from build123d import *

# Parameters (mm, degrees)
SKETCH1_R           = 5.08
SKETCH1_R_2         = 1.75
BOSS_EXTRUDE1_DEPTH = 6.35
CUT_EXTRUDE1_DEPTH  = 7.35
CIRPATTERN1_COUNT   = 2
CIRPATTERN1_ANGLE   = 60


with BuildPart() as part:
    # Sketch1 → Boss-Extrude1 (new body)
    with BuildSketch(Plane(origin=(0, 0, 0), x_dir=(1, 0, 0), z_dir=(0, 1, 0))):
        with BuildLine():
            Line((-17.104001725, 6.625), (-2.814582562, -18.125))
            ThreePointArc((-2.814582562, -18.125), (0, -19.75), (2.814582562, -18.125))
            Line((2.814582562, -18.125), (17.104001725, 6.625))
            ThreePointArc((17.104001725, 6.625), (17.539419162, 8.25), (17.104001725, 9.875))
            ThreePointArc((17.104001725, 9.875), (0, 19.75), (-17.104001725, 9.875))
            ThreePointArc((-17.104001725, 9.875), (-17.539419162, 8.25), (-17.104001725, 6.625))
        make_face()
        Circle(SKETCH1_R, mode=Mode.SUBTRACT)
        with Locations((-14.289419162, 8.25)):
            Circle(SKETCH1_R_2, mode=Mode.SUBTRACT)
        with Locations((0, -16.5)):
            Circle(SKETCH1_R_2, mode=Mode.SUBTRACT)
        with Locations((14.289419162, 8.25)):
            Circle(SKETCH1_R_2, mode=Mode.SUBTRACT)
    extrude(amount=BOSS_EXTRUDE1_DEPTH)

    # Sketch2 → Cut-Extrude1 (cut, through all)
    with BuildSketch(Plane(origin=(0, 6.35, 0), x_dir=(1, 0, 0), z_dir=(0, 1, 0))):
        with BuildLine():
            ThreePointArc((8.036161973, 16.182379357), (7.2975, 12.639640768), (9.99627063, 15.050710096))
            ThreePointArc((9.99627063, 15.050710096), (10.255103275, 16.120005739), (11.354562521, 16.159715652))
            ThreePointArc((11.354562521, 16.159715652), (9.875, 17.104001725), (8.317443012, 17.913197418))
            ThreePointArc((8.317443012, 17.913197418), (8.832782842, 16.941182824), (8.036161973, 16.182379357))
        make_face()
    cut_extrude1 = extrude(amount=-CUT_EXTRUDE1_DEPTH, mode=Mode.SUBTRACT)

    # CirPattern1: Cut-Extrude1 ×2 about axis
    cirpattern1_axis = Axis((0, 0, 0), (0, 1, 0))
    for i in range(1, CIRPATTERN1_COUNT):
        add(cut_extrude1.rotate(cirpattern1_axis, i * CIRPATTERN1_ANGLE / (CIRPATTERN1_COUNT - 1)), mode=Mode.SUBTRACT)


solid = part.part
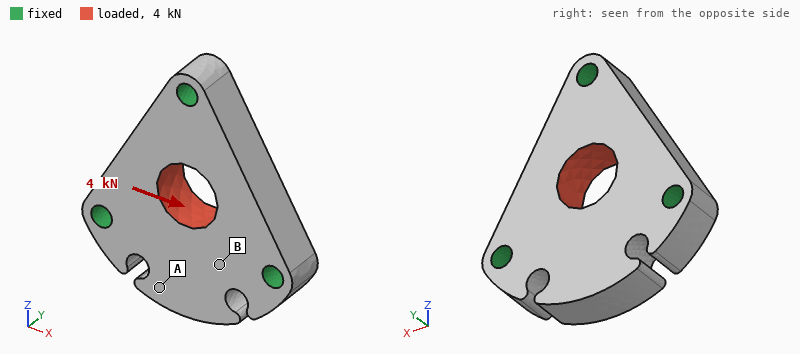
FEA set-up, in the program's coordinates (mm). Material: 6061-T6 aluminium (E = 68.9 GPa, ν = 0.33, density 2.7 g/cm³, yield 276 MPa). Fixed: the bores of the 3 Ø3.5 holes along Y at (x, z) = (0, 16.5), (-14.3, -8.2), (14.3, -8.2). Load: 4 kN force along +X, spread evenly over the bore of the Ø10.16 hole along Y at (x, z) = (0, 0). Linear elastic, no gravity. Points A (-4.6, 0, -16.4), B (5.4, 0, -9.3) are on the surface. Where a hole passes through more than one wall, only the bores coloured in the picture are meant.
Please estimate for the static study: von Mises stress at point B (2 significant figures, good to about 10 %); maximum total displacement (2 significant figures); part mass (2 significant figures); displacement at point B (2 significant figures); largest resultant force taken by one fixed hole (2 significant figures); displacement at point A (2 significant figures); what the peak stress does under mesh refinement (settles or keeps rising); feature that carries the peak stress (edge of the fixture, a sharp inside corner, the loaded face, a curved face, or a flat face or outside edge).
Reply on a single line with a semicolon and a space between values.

21 MPa; 12 µm; 12 g; 2.5 µm; 1.6 kN; 2.8 µm; keeps rising; edge of the fixture
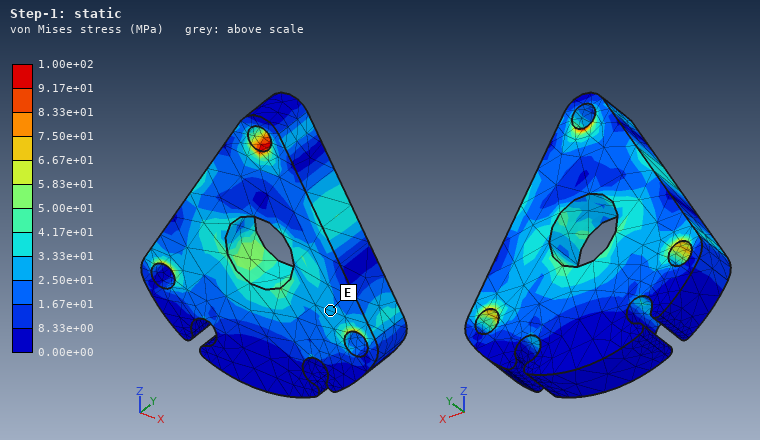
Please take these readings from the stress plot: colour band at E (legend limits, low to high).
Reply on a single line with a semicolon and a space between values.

2.50e+01 to 3.33e+01 MPa
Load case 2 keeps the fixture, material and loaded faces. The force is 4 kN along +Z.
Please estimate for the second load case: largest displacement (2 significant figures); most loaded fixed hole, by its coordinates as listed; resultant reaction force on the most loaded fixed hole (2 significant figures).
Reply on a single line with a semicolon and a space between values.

10 µm; (0, 16.5); 1.7 kN
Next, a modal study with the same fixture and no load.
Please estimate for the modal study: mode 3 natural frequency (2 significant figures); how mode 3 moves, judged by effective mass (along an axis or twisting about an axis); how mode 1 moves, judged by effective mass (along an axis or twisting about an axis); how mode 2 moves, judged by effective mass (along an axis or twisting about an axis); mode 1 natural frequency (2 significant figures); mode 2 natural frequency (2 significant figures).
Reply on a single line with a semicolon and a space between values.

36 kHz; along Z; along Y; along Y; 19 kHz; 32 kHz
